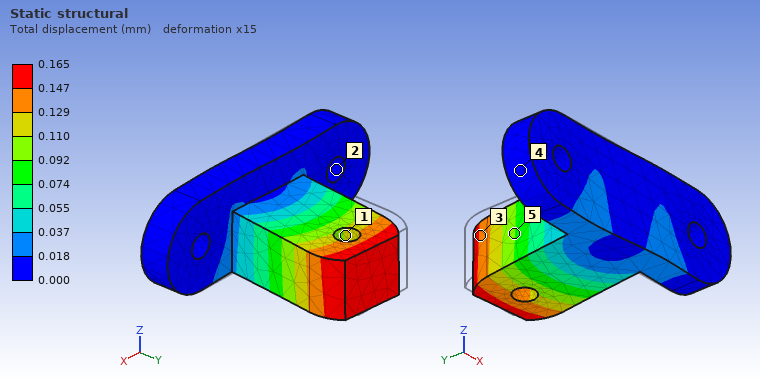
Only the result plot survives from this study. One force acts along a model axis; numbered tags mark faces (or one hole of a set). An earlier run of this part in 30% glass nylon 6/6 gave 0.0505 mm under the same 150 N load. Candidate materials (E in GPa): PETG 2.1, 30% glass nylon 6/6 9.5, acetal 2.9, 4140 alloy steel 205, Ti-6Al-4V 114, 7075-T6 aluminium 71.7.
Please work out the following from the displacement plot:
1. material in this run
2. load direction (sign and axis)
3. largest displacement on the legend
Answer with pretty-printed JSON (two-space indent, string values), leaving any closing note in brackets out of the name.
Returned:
{
  "material in this run": "acetal",
  "load direction": "+X",
  "largest displacement on the legend": "0.165 mm"
}
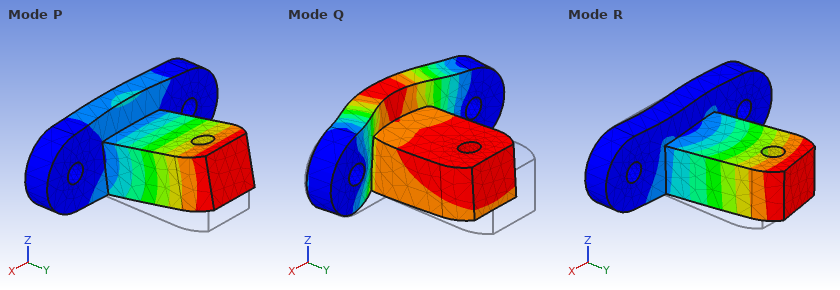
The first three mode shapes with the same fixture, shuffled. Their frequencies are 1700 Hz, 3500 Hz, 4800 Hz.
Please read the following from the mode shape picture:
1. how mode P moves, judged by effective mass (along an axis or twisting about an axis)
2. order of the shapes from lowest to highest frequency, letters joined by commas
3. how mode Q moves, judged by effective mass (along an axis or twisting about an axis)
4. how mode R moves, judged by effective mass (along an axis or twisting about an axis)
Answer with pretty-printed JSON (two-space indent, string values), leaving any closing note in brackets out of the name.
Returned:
{
  "how mode P moves, judged by effective mass": "along Z",
  "order of the shapes from lowest to highest frequency, letters joined by commas": "P, R, Q",
  "how mode Q moves, judged by effective mass": "along Y",
  "how mode R moves, judged by effective mass": "along X"
}
